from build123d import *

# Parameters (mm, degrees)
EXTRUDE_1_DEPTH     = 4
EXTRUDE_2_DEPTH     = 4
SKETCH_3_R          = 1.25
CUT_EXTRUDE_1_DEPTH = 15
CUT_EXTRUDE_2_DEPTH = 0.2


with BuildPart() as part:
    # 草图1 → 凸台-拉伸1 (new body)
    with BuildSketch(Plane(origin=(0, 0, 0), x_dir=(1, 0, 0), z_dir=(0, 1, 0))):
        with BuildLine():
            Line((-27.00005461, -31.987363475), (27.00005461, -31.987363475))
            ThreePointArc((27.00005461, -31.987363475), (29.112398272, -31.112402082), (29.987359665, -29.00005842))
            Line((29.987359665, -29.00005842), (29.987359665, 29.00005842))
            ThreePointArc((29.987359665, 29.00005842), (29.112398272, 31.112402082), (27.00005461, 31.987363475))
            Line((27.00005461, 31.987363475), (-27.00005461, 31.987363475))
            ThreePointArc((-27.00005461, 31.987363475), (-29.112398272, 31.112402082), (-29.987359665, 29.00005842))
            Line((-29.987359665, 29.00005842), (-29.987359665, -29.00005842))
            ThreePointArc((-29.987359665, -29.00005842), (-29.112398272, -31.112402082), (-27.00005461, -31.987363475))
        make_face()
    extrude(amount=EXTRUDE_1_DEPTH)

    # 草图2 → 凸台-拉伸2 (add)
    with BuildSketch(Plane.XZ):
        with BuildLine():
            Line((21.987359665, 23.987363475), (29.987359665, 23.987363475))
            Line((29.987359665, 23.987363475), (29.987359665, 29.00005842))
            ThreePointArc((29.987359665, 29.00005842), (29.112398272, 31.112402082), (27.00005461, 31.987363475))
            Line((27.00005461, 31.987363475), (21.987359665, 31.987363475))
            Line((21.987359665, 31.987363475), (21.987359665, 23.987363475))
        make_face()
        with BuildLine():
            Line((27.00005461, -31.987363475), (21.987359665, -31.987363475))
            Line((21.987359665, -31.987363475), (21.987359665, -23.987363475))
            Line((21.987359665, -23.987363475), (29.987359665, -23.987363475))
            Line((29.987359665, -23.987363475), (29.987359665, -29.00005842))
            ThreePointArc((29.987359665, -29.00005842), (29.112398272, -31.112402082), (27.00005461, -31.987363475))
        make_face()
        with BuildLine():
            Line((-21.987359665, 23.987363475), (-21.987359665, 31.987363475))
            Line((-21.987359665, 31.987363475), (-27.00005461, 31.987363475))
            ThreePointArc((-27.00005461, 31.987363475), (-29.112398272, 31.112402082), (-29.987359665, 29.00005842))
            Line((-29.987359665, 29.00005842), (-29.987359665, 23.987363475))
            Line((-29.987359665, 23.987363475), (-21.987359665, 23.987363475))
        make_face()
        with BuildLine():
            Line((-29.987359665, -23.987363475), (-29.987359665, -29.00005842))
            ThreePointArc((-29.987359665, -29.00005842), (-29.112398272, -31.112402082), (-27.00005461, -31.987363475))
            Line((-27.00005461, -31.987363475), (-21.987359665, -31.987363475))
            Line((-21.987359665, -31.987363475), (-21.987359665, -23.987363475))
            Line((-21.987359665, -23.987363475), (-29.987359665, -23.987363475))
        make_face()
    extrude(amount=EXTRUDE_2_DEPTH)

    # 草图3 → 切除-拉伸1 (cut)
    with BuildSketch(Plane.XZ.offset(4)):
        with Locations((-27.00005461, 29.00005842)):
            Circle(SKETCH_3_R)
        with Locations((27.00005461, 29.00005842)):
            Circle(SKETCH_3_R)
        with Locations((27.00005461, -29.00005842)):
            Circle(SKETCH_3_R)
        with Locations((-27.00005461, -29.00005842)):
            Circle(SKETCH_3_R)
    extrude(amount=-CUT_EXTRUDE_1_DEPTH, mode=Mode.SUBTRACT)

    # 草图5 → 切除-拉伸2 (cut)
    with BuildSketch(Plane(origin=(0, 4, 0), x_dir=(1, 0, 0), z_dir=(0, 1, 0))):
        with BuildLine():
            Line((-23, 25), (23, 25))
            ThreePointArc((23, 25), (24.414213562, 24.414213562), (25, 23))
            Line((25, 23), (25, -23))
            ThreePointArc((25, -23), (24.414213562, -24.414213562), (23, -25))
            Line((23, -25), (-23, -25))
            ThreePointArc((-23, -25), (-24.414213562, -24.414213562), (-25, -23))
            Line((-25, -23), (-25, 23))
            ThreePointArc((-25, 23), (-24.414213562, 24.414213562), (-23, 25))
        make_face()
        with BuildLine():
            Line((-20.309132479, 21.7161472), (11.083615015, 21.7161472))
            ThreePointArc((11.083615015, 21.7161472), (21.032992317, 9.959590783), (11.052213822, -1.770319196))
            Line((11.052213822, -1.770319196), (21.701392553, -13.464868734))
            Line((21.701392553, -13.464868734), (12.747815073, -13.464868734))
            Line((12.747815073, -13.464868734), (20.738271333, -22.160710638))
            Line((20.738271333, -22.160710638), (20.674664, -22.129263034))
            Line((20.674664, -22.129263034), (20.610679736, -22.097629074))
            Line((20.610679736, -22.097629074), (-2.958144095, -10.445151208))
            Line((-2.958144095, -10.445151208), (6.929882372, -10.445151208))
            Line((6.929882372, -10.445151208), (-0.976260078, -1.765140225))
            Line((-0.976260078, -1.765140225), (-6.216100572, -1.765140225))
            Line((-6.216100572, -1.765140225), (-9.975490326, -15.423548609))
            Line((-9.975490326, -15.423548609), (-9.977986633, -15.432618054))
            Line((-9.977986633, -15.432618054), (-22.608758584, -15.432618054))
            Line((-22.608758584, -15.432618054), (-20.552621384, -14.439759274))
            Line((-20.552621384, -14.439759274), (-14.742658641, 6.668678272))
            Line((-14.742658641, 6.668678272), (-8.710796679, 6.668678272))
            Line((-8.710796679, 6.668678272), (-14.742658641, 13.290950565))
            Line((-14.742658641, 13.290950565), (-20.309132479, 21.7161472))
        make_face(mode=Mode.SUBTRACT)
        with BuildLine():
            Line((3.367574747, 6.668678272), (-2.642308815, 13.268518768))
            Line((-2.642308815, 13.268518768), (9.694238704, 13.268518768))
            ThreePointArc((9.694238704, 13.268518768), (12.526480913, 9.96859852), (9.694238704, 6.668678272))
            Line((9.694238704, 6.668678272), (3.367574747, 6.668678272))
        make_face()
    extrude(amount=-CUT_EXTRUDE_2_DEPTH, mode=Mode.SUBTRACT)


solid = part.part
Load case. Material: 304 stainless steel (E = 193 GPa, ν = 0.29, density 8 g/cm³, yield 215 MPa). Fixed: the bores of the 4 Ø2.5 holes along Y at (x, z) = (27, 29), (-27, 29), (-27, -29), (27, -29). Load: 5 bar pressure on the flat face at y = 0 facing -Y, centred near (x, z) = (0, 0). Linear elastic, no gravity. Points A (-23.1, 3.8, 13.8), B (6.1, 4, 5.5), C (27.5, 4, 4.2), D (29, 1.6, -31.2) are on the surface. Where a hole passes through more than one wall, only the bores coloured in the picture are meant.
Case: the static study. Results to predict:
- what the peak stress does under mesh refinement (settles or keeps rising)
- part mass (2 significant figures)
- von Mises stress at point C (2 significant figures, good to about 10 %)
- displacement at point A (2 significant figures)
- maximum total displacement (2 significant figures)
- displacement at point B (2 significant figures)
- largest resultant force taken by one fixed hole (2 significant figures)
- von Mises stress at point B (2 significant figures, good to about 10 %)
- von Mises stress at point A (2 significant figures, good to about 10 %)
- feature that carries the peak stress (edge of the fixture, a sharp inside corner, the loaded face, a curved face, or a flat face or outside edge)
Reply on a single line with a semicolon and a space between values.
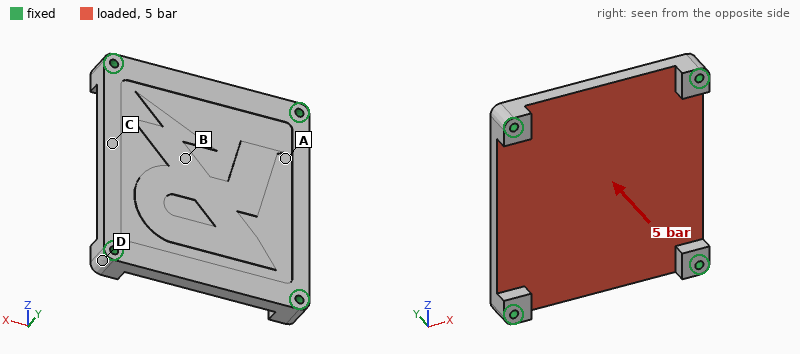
keeps rising; 130 g; 34 MPa; 12 µm; 29 µm; 27 µm; 500 N; 28 MPa; 14 MPa; edge of the fixture
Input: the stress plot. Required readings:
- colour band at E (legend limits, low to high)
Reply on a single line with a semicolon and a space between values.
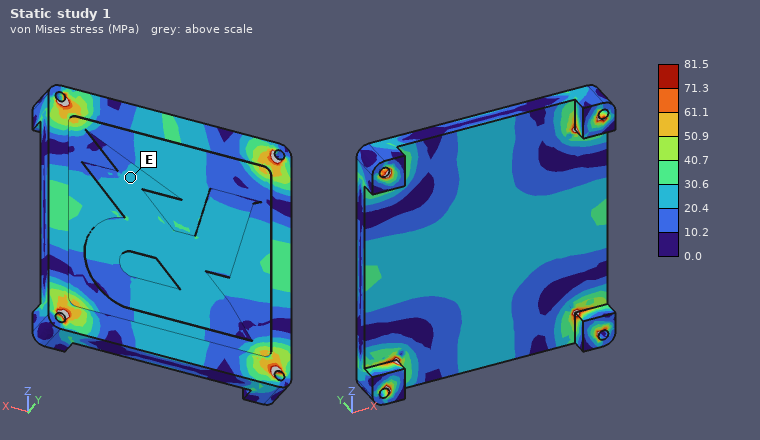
20.4 to 30.6 MPa
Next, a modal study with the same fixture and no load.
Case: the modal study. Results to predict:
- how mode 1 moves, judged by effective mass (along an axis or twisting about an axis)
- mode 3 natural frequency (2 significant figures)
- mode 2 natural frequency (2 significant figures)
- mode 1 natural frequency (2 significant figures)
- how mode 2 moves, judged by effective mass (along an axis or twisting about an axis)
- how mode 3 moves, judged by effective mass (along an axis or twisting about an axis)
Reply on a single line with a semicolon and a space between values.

along Y; 8100 Hz; 7400 Hz; 4500 Hz; twisting about Z; twisting about X
